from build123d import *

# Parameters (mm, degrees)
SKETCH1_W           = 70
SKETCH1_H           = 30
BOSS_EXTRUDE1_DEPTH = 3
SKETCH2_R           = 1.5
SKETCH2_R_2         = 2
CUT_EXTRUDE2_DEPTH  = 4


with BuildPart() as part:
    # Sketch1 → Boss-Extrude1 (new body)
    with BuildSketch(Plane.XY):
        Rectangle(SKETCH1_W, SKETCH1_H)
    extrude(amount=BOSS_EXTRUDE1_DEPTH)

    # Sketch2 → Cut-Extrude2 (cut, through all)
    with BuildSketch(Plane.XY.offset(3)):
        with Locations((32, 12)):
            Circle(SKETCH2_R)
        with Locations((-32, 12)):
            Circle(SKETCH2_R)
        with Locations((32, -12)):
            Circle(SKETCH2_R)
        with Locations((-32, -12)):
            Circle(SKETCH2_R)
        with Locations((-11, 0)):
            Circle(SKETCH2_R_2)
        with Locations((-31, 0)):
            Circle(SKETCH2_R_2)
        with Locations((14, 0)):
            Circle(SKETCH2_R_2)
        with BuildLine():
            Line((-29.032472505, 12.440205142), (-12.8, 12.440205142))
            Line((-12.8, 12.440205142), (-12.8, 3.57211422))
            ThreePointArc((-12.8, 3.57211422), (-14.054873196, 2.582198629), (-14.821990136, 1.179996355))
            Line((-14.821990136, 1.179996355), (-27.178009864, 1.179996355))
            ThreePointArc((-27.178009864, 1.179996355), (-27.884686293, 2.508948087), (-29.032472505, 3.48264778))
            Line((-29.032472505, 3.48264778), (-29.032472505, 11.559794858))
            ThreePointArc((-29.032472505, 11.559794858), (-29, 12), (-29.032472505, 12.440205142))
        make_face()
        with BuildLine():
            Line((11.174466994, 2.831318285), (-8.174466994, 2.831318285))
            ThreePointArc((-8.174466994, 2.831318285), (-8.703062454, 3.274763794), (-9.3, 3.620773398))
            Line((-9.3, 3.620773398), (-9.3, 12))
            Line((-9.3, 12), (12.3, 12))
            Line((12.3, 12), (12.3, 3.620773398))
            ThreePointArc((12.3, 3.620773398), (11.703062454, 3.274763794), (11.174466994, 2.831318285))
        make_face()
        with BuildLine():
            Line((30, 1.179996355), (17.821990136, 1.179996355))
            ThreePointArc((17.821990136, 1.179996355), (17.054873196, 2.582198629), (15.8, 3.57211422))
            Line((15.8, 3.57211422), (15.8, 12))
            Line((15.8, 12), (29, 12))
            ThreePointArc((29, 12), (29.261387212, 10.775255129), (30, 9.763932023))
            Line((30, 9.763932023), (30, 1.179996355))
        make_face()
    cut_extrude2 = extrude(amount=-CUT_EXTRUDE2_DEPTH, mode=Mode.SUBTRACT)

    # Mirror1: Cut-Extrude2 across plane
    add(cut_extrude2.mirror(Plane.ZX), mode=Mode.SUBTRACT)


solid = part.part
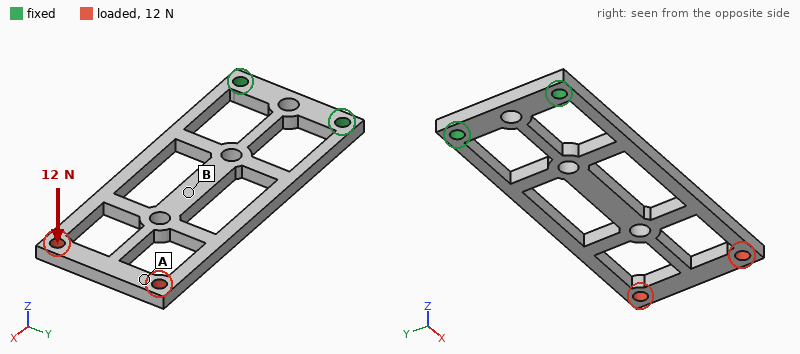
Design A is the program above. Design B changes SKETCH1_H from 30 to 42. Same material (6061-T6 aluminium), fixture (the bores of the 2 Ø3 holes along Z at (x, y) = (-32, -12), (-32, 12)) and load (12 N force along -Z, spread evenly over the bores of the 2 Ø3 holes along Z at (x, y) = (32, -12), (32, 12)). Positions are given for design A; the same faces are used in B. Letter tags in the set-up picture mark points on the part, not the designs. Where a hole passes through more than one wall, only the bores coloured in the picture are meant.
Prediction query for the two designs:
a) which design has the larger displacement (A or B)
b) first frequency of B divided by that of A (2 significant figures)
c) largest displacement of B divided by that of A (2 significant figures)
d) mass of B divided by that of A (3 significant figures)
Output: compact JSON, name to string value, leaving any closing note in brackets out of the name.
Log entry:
{"which design has the larger displacement": "A", "first frequency of B divided by that of A": "1.1", "largest displacement of B divided by that of A": "0.44", "mass of B divided by that of A": "1.85"}
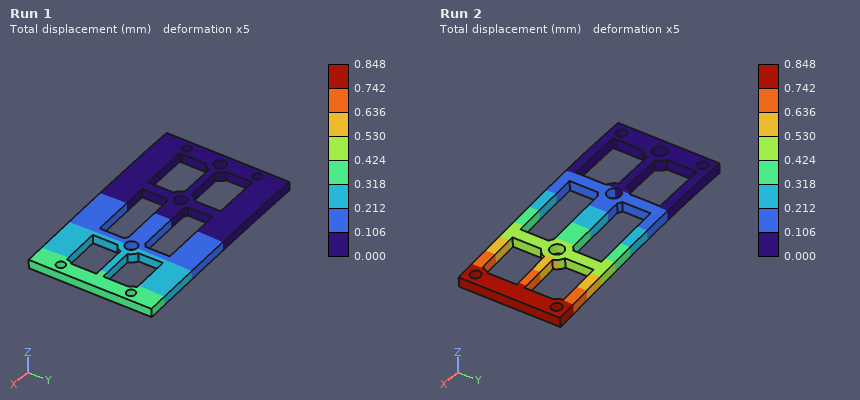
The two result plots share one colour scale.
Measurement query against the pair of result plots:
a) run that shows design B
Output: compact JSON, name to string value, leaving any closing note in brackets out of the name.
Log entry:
{"run that shows design B": "Run 1"}
